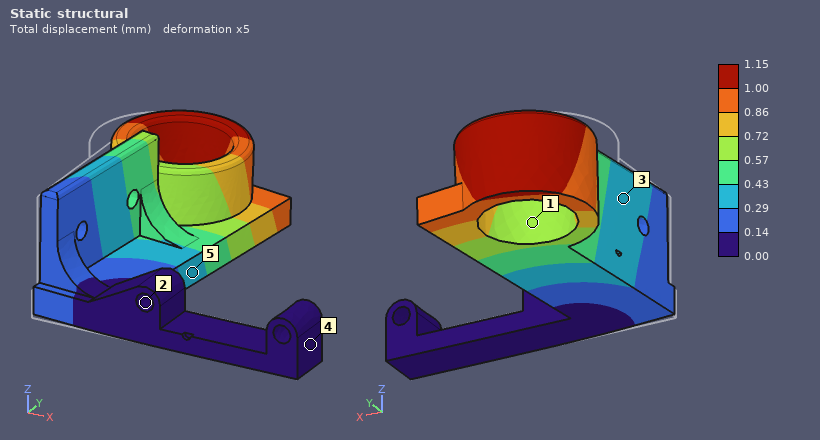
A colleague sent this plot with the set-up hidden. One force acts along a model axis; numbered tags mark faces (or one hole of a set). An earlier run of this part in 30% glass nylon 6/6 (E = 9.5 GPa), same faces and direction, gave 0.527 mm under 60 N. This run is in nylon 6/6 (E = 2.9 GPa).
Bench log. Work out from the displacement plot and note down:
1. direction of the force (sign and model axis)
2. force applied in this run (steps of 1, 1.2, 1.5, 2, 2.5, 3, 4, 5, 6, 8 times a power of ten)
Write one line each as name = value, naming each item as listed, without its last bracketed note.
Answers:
direction of the force = +X
force applied in this run = 40 N
